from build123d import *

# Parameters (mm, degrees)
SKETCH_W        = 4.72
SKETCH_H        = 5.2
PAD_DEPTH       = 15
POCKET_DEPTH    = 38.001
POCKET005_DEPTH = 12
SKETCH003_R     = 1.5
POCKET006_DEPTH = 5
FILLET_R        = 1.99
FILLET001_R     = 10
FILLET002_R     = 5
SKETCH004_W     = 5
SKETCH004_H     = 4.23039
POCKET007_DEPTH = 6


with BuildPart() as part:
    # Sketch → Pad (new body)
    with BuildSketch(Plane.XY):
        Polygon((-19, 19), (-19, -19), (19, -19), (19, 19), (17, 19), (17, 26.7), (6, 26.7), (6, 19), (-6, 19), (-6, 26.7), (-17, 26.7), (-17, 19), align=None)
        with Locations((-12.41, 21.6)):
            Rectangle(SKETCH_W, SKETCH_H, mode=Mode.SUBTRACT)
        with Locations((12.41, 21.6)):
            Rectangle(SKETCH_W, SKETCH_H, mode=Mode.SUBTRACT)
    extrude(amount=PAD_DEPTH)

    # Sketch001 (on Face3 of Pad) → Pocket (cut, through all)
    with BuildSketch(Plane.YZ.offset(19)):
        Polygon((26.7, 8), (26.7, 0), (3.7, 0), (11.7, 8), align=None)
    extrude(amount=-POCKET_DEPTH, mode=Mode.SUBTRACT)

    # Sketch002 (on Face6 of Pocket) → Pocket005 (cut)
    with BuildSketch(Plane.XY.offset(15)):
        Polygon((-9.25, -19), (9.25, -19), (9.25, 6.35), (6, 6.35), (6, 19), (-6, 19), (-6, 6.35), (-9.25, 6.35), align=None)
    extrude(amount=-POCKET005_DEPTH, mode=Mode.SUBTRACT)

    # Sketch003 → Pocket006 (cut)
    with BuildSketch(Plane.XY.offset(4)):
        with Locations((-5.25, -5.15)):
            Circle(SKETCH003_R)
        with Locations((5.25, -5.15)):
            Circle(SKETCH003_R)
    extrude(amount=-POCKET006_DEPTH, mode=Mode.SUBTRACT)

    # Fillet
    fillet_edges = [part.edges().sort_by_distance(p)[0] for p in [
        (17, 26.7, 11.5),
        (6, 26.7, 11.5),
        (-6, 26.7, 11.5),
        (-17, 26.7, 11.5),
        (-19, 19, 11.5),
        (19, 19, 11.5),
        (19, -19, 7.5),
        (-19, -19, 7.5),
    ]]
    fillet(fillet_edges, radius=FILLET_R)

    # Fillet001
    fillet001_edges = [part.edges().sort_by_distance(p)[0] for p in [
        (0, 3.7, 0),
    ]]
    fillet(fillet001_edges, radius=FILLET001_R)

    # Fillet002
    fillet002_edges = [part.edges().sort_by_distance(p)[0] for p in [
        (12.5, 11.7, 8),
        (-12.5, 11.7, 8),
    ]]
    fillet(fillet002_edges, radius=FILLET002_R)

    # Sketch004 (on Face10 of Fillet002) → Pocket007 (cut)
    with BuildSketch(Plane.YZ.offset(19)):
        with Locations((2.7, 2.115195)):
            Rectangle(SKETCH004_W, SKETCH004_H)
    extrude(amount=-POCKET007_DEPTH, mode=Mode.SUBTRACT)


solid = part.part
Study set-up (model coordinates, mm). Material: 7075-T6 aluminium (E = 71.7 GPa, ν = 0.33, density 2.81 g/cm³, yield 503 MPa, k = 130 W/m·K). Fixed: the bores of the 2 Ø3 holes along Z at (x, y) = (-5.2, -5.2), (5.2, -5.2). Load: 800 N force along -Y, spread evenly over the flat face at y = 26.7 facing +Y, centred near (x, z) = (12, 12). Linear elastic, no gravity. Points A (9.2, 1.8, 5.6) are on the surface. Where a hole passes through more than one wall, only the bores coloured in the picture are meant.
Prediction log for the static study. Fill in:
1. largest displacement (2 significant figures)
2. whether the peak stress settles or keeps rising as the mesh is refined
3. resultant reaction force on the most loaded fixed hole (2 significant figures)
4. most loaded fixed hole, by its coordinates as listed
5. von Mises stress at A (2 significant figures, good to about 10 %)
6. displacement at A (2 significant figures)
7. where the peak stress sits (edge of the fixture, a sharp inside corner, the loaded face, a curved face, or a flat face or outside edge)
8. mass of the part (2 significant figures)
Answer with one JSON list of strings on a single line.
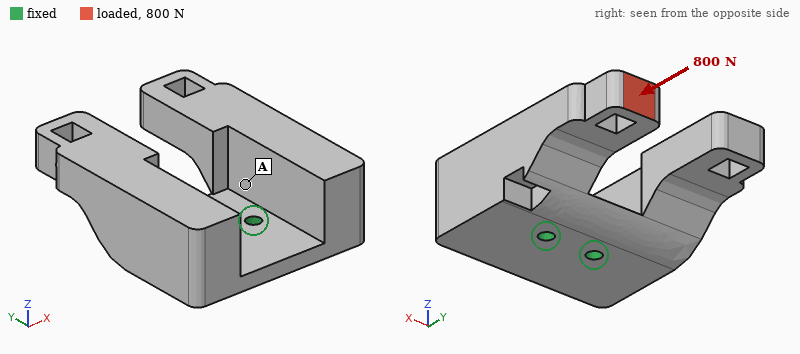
["0.24 mm", "keeps rising", "1.1 kN", "(5.2, -5.2)", "39 MPa", "0.055 mm", "edge of the fixture", "34 g"]
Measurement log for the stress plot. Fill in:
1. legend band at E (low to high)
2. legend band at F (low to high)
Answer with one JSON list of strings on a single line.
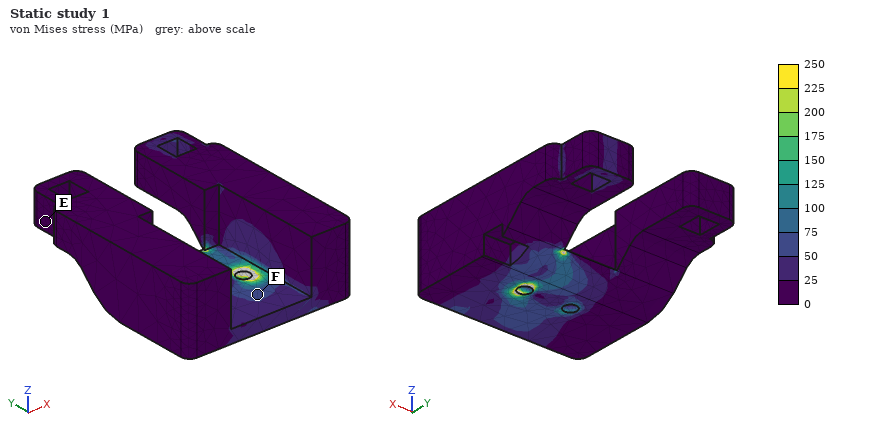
["0 to 25 MPa", "50 to 75 MPa"]
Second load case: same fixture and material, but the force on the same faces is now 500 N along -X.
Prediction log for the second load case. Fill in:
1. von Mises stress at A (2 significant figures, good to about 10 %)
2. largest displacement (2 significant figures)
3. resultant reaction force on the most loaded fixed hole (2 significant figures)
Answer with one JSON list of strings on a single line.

["64 MPa", "0.26 mm", "1.2 kN"]
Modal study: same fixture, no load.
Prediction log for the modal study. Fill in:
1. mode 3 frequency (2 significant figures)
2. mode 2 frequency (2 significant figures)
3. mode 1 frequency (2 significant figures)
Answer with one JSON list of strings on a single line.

["3100 Hz", "3000 Hz", "2600 Hz"]
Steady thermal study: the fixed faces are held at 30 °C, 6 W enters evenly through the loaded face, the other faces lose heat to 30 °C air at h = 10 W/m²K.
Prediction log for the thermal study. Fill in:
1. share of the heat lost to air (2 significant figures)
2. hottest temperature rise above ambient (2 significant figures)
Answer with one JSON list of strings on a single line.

["4.3 %", "25 K"]
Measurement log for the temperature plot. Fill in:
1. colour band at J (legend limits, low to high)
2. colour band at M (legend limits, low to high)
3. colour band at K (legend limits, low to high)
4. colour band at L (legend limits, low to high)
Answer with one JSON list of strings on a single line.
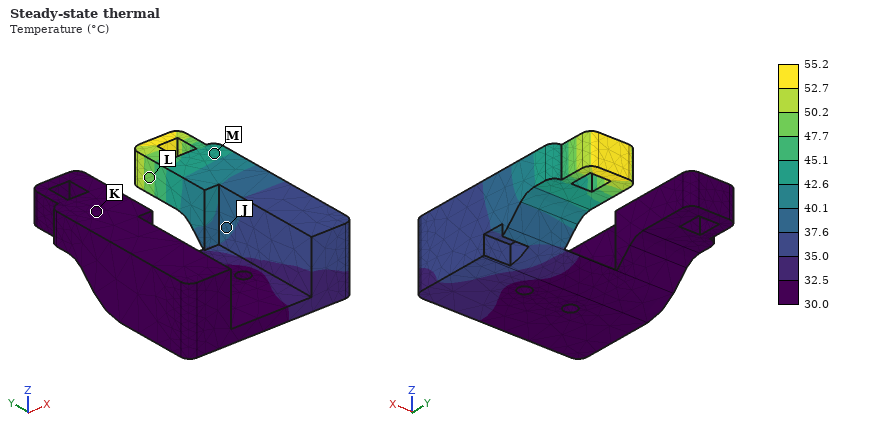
["37.6 to 40.1 °C", "42.6 to 45.1 °C", "30.0 to 32.5 °C", "47.7 to 50.2 °C"]
